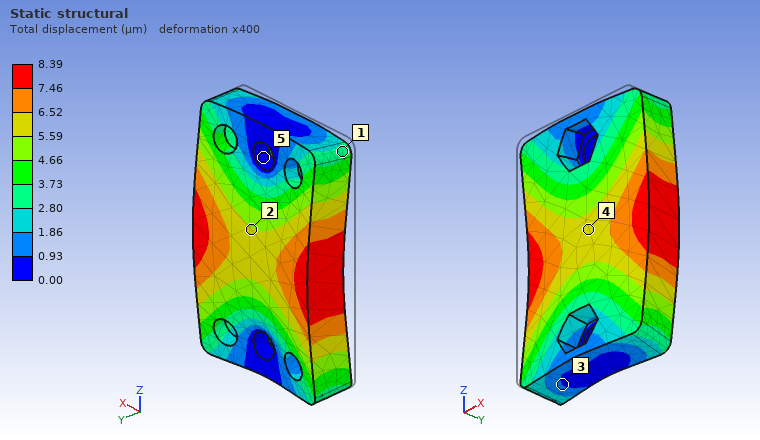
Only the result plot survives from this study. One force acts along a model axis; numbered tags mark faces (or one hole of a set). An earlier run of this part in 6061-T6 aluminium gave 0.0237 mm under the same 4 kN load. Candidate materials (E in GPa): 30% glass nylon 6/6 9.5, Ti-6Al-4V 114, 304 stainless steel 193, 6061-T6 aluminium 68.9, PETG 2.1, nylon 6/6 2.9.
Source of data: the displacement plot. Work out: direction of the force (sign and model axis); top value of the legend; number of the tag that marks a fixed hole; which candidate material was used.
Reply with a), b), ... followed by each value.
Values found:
a) +Y
b) 8.39 µm
c) 5
d) 304 stainless steel
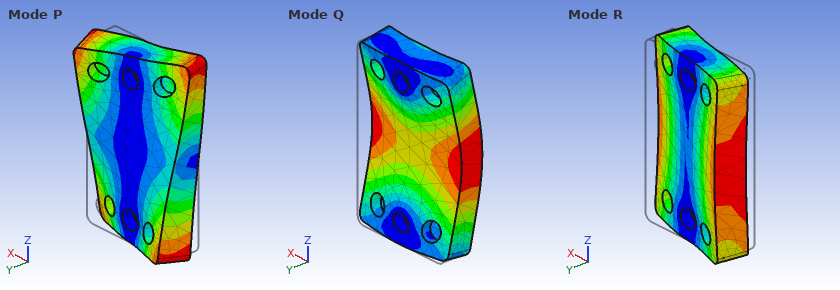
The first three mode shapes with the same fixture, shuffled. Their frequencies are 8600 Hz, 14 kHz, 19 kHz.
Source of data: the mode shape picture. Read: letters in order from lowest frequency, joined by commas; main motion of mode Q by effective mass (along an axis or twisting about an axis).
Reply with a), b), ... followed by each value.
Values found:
a) R, Q, P
b) along Y
